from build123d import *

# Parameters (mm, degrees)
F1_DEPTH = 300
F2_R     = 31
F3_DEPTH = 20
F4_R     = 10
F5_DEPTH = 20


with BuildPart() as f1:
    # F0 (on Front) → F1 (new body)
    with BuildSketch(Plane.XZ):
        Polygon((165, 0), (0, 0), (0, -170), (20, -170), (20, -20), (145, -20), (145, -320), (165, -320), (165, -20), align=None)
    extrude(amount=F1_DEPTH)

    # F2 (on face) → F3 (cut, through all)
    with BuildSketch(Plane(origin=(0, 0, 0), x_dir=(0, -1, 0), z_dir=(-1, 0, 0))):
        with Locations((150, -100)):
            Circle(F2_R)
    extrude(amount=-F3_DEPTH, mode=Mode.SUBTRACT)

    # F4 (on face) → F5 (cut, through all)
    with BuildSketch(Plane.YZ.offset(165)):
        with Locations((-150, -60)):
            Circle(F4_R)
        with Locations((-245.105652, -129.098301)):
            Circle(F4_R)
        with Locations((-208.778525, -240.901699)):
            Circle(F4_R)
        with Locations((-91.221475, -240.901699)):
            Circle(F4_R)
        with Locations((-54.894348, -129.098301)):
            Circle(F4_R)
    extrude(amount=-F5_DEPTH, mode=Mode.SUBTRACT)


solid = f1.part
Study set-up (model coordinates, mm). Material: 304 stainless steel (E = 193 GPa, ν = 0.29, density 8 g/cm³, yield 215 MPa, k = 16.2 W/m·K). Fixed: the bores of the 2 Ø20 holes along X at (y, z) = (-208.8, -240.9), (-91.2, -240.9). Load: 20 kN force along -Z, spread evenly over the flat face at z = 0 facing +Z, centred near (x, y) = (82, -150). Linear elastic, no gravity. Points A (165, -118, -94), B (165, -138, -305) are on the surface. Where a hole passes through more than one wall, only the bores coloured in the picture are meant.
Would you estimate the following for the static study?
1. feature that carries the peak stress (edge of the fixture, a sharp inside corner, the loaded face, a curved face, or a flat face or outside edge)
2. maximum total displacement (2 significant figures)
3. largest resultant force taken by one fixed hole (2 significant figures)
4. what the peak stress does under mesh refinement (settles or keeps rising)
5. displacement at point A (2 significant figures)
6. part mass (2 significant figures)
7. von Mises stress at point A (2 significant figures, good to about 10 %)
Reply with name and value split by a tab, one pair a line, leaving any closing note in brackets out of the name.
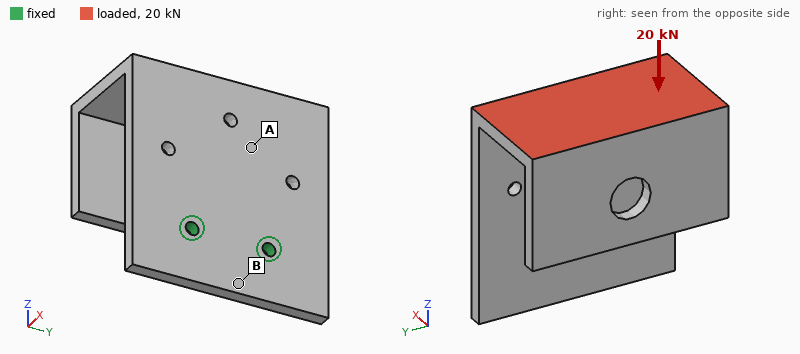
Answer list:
feature that carries the peak stress	edge of the fixture
maximum total displacement	1.9 mm
largest resultant force taken by one fixed hole	10 kN
what the peak stress does under mesh refinement	keeps rising
displacement at point A	0.45 mm
part mass	29 kg
von Mises stress at point A	63 MPa
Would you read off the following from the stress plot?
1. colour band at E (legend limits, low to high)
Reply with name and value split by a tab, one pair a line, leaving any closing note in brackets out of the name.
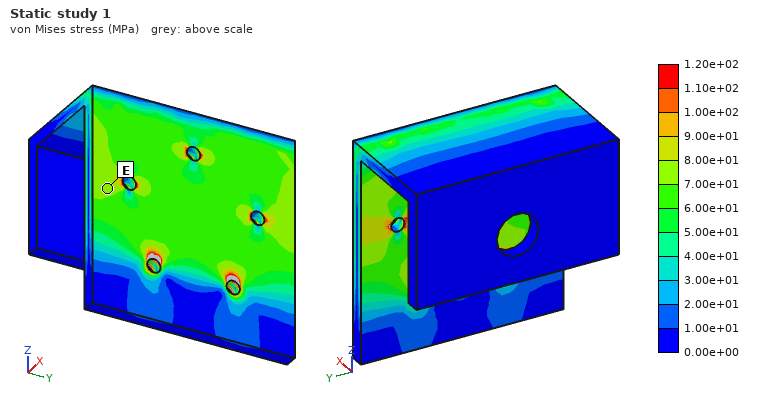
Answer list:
colour band at E	7.00e+01 to 8.00e+01 MPa
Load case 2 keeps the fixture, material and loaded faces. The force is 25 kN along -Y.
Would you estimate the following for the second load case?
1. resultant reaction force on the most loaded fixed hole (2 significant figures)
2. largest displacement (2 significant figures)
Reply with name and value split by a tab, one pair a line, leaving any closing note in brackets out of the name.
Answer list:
resultant reaction force on the most loaded fixed hole	49 kN
largest displacement	1.1 mm
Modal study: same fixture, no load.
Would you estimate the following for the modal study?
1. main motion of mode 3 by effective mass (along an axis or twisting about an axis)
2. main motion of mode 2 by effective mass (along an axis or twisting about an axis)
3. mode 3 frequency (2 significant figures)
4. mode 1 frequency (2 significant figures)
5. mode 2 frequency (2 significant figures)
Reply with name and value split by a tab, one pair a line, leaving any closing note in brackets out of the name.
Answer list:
main motion of mode 3 by effective mass	along X
main motion of mode 2 by effective mass	along Y
mode 3 frequency	200 Hz
mode 1 frequency	100 Hz
mode 2 frequency	160 Hz
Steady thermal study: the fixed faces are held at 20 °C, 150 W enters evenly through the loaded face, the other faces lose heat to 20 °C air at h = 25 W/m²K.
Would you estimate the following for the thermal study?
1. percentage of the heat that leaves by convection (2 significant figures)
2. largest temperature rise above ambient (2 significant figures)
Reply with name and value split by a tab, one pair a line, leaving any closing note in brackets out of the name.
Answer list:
percentage of the heat that leaves by convection	98 %
largest temperature rise above ambient	54 K
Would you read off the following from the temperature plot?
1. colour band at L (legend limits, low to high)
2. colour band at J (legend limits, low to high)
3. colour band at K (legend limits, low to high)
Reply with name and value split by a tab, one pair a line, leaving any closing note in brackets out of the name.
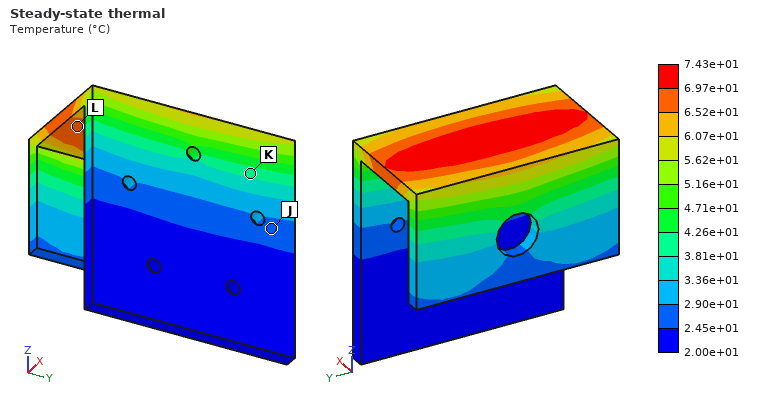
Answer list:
colour band at L	6.52e+01 to 6.97e+01 °C
colour band at J	2.45e+01 to 2.90e+01 °C
colour band at K	3.81e+01 to 4.26e+01 °C
